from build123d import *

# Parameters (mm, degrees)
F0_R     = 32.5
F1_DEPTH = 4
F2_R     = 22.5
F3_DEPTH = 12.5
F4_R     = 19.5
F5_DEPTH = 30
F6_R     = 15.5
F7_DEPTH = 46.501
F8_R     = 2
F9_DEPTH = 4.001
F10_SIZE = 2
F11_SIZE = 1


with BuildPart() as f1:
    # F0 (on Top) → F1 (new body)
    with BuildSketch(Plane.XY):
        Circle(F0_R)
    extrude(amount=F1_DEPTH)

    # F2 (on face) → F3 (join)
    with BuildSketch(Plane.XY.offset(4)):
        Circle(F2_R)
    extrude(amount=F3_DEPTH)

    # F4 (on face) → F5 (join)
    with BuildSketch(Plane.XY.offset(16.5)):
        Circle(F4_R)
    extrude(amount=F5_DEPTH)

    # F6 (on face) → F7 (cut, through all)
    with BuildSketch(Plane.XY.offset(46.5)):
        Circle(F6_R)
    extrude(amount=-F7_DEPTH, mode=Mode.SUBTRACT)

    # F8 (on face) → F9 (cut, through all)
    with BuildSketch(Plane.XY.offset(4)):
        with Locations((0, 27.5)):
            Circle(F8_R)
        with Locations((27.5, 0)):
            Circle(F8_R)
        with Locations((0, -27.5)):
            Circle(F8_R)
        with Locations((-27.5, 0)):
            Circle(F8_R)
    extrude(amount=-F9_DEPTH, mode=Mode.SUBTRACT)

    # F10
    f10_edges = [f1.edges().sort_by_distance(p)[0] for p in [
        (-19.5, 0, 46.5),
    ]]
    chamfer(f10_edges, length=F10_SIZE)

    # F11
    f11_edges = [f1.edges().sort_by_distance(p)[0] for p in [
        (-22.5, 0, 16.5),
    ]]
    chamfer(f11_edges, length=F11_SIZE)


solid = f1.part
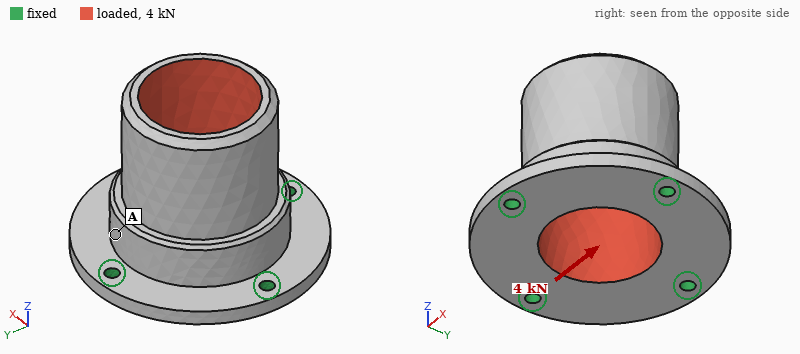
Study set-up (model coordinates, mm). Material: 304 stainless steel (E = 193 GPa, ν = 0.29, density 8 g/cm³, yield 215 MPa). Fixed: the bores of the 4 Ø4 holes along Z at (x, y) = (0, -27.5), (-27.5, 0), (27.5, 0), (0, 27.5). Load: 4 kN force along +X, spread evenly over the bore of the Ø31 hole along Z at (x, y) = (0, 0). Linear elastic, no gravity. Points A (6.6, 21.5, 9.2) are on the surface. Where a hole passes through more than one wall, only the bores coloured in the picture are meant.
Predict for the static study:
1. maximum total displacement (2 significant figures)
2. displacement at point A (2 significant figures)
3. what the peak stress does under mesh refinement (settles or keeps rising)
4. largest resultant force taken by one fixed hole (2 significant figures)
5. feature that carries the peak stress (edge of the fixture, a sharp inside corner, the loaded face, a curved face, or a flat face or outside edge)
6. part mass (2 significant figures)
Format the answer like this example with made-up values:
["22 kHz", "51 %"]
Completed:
["17 µm", "3.4 µm", "keeps rising", "2.1 kN", "edge of the fixture", "270 g"]
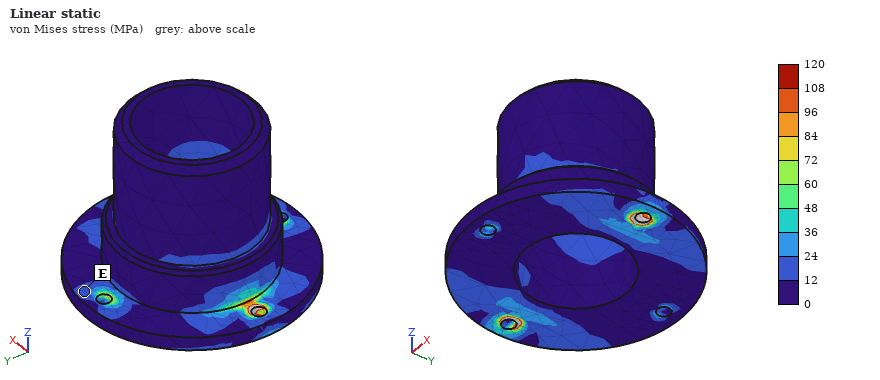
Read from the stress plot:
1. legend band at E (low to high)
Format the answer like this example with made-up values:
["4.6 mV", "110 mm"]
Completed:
["12 to 24 MPa"]
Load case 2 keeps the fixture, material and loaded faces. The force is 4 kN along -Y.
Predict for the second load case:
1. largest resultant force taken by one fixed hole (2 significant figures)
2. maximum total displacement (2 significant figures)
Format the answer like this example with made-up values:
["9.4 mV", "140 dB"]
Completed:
["2.1 kN", "17 µm"]
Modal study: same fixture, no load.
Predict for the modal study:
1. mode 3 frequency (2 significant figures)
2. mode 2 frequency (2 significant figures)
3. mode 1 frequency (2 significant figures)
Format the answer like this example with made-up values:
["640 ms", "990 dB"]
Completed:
["9300 Hz", "6700 Hz", "6700 Hz"]
